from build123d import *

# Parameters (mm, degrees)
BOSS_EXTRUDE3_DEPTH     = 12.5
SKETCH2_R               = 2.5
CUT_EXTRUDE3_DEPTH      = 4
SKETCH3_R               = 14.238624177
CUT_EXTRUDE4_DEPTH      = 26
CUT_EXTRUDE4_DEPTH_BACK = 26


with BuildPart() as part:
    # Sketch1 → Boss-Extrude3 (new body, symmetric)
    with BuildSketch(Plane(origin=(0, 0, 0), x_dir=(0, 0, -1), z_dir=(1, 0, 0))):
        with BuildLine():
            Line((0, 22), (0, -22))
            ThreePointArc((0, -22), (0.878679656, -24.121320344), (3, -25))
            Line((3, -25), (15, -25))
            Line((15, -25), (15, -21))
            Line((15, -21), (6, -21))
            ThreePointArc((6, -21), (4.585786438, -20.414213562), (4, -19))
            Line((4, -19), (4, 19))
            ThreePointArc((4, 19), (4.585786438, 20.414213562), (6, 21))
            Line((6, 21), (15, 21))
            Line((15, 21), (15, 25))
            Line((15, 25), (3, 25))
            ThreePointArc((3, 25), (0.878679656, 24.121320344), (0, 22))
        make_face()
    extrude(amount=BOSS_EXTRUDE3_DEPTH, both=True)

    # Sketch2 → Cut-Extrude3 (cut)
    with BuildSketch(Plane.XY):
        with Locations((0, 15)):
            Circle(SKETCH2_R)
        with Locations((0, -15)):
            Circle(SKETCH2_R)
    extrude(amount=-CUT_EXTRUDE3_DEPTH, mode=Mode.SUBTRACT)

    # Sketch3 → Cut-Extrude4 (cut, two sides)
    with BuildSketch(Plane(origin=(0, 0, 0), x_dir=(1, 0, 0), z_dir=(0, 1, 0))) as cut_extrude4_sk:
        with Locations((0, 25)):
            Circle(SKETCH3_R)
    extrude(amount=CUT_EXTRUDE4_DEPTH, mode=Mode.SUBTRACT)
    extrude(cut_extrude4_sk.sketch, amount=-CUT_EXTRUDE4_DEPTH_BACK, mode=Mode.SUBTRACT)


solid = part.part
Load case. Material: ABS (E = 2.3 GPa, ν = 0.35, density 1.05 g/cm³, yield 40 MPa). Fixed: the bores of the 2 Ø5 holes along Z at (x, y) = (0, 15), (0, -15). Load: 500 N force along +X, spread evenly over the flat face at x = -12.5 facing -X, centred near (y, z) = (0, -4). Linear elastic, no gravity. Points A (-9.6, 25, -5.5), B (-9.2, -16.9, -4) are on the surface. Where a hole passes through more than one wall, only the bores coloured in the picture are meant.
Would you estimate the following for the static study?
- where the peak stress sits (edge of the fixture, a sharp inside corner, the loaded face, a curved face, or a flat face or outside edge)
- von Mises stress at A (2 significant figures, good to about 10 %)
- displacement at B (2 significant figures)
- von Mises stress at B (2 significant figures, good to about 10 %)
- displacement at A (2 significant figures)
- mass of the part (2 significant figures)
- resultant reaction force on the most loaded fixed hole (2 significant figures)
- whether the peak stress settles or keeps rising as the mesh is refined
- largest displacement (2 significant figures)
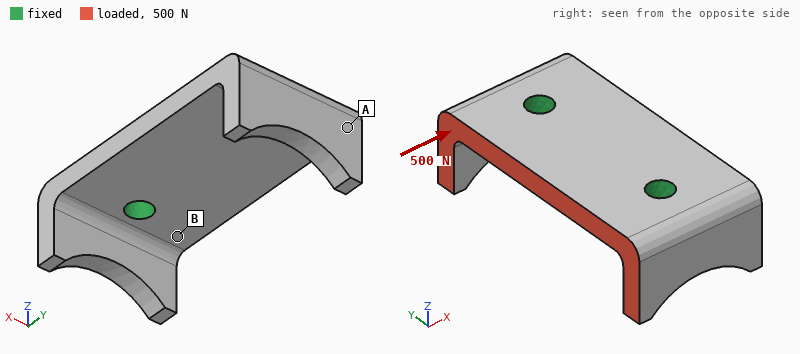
edge of the fixture
2.2 MPa
0.049 mm
4.3 MPa
0.091 mm
6.8 g
250 N
keeps rising
0.18 mm
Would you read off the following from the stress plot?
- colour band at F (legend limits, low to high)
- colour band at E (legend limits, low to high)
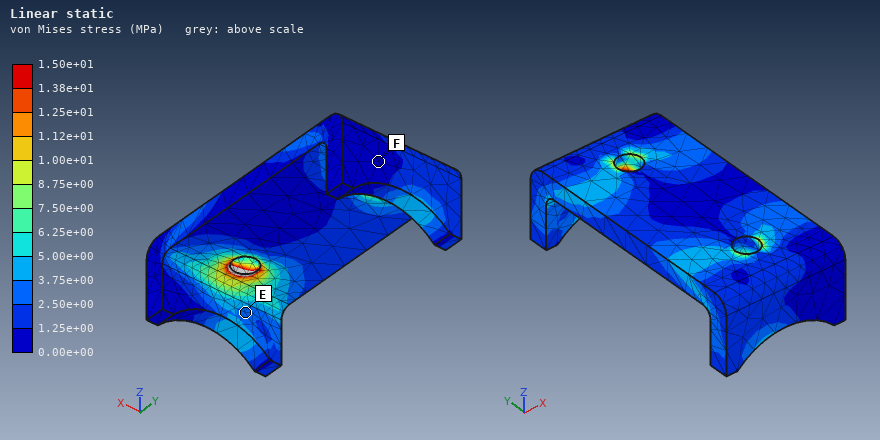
0.00e+00 to 1.25e+00 MPa
2.50e+00 to 3.75e+00 MPa
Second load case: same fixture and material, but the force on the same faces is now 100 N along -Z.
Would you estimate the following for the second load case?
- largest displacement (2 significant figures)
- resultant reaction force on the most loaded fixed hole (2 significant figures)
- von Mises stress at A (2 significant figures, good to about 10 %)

0.12 mm
50 N
1.4 MPa
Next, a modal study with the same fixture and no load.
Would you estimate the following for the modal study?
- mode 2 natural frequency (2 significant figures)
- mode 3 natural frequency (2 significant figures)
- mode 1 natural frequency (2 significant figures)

3700 Hz
3700 Hz
3600 Hz
